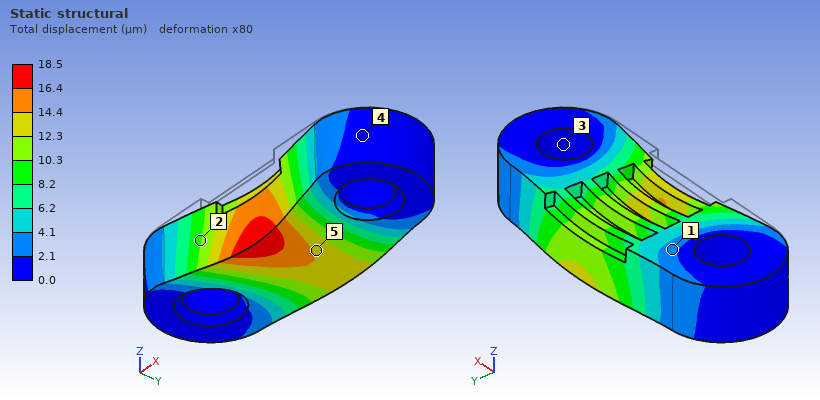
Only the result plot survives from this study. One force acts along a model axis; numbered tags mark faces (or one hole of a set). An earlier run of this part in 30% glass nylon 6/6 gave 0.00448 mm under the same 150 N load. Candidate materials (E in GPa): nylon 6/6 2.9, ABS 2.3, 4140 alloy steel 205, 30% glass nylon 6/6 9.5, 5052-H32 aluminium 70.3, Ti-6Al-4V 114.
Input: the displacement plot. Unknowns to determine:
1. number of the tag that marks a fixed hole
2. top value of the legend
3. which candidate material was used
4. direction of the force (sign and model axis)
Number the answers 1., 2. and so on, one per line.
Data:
1. 3
2. 18.5 µm
3. ABS
4. +Y
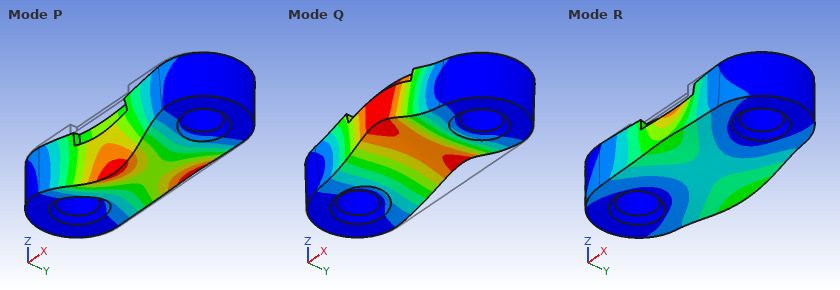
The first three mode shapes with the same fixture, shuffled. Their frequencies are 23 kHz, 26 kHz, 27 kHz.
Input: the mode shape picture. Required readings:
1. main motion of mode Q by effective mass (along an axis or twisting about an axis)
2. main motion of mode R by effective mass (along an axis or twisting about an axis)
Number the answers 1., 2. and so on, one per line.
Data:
1. along Z
2. along Y
